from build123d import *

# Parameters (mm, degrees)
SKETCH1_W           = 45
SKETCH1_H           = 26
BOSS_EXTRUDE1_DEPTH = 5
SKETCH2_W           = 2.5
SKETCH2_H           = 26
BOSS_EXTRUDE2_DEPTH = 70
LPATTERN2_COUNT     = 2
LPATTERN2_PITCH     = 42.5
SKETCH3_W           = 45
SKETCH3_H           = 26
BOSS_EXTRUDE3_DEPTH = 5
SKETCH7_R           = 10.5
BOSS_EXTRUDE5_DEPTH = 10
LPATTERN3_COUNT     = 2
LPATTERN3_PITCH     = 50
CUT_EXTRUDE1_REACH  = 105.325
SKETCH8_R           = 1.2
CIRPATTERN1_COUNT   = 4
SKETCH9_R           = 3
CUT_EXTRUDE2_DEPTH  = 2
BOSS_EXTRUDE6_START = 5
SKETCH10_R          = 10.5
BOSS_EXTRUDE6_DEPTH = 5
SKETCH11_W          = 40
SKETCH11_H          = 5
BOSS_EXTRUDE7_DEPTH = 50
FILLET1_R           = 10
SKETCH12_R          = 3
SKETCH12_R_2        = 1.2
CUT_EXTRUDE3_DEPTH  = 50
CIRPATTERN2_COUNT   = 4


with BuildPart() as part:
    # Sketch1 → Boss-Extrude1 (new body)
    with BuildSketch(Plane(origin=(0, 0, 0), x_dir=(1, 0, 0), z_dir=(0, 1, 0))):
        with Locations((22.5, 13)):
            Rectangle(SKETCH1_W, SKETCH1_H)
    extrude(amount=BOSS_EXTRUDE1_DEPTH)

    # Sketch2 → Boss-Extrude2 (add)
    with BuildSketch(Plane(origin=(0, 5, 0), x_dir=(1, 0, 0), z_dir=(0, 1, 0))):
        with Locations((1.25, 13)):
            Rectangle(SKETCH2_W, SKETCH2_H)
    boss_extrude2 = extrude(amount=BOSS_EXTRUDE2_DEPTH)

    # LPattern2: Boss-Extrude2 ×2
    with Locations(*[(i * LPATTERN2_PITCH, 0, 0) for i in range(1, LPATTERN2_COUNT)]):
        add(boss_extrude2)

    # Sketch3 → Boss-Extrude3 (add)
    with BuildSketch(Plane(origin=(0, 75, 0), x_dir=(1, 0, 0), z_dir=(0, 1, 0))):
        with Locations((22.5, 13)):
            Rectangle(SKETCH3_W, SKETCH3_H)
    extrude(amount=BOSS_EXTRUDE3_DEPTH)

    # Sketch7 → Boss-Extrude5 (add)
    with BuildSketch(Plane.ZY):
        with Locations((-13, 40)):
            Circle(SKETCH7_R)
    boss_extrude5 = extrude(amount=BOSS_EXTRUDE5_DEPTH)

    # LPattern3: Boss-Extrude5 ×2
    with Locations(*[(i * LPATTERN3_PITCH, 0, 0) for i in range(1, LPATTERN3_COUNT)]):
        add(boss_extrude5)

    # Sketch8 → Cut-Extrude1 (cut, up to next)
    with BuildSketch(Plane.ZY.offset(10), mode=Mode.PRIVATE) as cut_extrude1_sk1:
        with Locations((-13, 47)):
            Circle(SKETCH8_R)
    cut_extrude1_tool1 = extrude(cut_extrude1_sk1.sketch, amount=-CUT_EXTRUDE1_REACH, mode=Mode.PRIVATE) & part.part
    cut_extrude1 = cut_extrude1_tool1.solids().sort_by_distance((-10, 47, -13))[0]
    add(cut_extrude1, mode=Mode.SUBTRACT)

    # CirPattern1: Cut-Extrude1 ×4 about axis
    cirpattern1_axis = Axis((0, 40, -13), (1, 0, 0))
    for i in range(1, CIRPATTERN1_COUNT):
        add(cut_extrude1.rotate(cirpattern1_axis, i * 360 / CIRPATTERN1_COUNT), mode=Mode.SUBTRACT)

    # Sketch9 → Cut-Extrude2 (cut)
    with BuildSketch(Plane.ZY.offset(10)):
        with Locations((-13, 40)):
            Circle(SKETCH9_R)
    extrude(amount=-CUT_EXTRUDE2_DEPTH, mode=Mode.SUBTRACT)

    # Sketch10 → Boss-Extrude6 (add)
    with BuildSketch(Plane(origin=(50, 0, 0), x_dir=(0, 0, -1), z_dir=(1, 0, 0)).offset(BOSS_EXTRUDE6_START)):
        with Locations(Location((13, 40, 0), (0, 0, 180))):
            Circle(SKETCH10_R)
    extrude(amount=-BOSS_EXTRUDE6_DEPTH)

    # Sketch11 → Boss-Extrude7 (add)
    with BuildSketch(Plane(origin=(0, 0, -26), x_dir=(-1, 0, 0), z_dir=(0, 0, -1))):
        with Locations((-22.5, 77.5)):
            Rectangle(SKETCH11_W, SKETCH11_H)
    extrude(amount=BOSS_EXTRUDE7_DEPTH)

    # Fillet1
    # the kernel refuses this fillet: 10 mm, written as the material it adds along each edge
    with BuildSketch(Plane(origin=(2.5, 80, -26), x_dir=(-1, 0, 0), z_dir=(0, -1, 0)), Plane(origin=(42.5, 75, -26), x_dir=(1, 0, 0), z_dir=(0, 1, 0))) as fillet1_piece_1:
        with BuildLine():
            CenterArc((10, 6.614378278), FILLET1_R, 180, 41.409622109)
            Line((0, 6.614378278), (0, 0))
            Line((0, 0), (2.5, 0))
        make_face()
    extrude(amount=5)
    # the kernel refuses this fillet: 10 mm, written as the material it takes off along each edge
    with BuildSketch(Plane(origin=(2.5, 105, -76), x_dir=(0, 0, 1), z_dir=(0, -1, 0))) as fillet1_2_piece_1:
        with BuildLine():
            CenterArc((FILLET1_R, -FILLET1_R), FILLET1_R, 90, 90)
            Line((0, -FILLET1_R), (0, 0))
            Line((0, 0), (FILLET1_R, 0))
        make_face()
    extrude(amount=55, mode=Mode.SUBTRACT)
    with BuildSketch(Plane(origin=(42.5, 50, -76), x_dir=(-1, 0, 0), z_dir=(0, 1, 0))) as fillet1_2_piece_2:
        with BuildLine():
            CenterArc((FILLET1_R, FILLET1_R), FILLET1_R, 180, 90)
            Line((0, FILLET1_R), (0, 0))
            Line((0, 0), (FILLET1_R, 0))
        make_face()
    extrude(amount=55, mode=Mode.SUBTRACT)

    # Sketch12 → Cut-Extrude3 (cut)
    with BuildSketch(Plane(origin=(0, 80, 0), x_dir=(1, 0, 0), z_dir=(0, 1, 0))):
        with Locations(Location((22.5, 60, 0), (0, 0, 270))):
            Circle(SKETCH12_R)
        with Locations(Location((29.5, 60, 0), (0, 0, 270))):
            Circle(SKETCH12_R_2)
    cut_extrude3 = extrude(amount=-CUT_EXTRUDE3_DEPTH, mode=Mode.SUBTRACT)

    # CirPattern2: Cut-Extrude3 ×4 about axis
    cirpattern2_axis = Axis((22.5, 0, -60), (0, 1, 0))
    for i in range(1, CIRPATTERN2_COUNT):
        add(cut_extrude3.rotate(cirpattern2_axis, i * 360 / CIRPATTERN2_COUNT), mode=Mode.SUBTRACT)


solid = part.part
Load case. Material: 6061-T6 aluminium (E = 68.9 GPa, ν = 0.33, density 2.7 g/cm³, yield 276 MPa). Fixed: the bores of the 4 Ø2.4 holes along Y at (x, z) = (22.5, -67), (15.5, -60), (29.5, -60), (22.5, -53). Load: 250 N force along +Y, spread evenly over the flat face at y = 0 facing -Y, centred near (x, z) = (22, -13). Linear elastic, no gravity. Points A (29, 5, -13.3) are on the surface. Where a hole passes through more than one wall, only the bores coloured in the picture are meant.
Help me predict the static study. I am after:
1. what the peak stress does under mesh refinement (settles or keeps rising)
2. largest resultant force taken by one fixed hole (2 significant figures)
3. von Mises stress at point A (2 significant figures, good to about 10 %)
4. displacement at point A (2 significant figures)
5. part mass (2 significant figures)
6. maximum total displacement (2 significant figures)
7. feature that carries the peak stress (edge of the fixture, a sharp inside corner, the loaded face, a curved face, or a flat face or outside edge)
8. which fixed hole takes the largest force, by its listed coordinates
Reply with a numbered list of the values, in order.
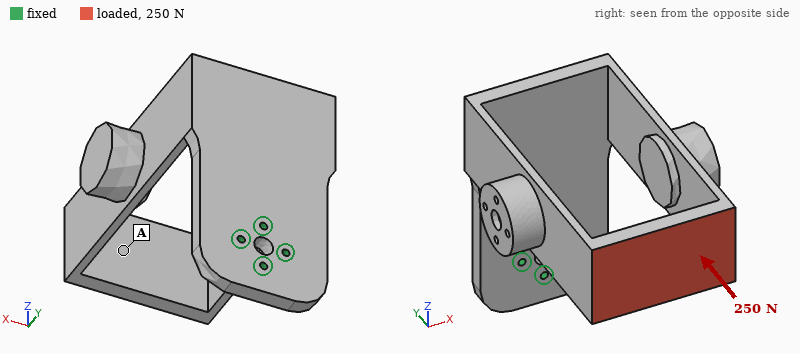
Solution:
1. keeps rising
2. 730 N
3. 8.9 MPa
4. 0.58 mm
5. 100 g
6. 0.66 mm
7. edge of the fixture
8. (22.5, -53)
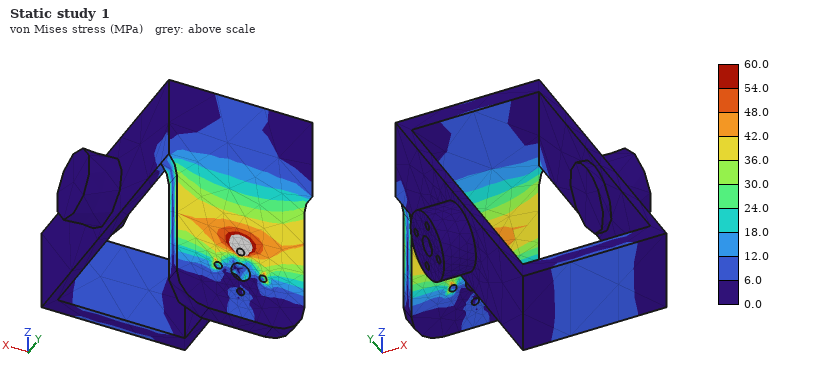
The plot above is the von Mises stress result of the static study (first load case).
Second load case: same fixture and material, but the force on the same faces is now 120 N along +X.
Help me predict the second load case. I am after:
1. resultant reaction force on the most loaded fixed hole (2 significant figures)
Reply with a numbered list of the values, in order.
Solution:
1. 360 N
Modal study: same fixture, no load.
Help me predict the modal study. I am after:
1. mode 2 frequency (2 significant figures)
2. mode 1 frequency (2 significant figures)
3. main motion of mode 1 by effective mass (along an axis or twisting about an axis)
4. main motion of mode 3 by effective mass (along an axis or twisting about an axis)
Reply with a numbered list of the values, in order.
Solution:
1. 300 Hz
2. 280 Hz
3. along X
4. twisting about Y
